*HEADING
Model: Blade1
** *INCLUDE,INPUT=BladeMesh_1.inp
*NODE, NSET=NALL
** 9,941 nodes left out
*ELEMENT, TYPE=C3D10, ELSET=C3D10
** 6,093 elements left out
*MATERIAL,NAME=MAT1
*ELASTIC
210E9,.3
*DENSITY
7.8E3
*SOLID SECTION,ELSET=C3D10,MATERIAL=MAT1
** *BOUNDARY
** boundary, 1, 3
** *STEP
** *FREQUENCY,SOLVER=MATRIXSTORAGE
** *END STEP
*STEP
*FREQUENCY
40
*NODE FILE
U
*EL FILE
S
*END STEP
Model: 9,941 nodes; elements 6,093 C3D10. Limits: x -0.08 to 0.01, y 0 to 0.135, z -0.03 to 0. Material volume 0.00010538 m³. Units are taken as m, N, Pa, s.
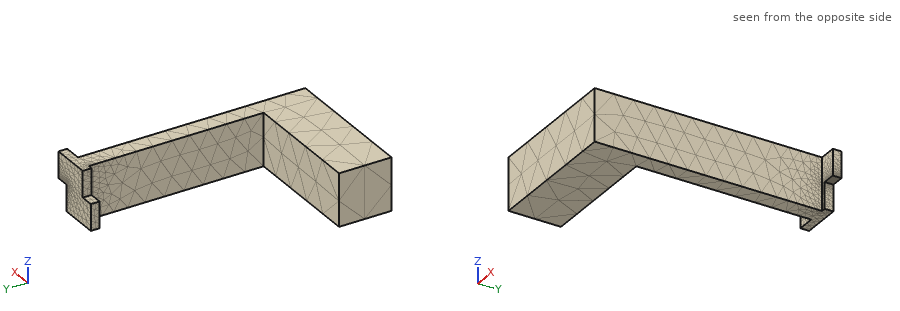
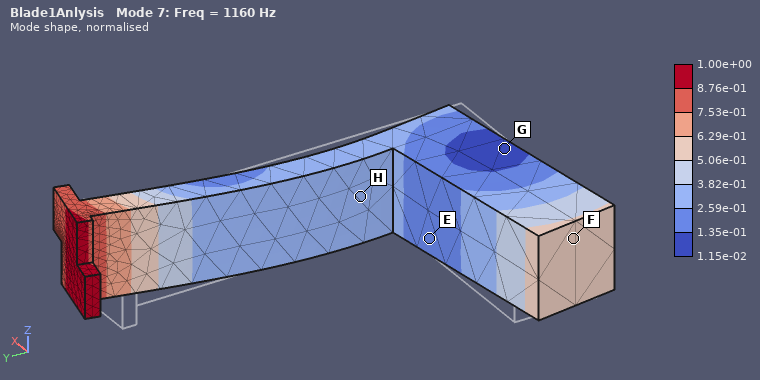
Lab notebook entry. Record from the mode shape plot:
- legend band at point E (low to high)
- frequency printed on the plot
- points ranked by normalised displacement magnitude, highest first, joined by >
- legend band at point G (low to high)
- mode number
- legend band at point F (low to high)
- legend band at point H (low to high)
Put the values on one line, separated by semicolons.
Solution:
1.35e-01 to 2.59e-01; 1160 Hz; F > H > E > G; 1.15e-02 to 1.35e-01; 7; 5.06e-01 to 6.29e-01; 2.59e-01 to 3.82e-01
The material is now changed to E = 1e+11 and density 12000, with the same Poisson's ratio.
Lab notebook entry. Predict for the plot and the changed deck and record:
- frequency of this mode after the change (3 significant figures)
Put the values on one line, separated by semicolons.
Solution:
645 Hz
